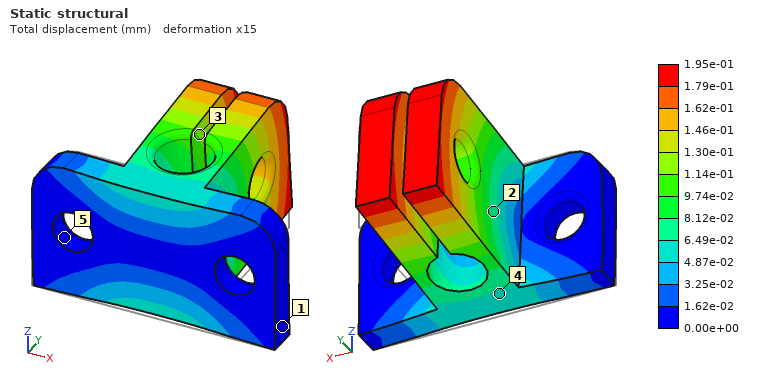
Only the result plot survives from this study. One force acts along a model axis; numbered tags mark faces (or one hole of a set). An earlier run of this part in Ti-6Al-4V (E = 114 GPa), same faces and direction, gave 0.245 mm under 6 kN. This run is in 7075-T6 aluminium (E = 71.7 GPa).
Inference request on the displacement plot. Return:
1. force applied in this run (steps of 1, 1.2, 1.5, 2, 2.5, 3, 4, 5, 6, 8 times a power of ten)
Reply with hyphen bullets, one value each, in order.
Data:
- 3 kN
